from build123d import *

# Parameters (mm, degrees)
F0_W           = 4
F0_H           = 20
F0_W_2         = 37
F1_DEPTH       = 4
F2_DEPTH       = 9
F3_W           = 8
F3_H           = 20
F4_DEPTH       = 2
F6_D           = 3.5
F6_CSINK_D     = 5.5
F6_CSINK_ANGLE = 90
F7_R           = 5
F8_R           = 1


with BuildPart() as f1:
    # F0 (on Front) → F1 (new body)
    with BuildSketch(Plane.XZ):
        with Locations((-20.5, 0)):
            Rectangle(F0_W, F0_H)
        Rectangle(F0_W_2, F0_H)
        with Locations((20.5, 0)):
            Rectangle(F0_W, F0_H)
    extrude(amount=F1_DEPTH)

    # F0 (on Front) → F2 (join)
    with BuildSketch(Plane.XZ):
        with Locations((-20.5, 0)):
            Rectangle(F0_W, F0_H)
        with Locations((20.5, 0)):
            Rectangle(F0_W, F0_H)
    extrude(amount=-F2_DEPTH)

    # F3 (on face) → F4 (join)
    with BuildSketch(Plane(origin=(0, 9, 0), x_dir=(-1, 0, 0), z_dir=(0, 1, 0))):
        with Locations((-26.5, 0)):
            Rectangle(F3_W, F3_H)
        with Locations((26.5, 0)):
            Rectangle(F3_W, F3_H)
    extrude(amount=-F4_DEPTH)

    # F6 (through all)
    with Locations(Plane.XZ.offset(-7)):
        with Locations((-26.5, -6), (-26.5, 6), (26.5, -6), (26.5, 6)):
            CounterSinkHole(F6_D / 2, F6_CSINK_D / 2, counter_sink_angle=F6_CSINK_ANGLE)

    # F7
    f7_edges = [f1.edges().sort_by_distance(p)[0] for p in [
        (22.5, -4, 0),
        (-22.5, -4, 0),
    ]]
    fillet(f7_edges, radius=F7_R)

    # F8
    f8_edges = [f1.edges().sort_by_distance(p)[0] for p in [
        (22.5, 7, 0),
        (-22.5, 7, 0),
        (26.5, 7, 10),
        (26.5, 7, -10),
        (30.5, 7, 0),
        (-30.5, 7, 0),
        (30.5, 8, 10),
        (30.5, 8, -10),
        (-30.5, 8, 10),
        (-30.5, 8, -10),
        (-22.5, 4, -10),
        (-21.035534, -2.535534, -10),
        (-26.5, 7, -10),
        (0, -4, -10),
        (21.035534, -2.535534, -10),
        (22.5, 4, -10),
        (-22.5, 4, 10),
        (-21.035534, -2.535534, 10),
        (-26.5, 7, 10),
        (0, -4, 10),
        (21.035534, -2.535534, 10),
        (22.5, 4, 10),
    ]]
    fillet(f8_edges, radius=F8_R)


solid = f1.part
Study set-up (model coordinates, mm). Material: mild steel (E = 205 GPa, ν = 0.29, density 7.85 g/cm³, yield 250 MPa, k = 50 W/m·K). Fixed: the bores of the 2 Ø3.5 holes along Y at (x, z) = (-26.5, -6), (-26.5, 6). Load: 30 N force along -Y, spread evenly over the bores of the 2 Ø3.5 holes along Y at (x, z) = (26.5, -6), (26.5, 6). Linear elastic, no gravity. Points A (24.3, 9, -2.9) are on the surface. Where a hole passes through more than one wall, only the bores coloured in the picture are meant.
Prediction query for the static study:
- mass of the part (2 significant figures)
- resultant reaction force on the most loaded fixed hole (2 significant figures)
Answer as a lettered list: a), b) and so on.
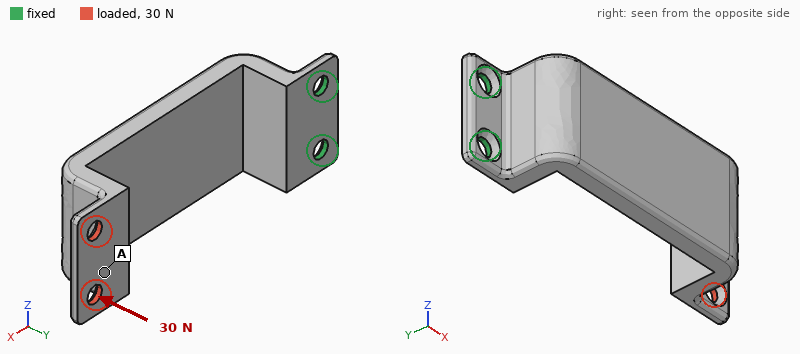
a) 42 g
b) 22 N
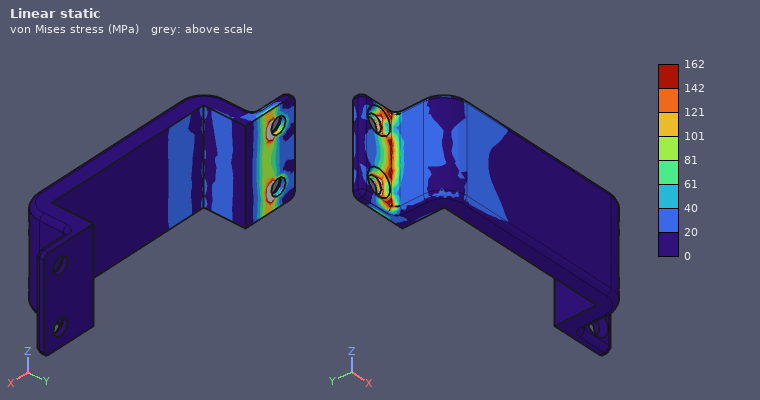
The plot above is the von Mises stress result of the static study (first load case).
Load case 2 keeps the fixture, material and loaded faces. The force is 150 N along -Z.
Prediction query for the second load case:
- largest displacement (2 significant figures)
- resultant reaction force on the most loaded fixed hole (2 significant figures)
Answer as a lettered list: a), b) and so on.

a) 0.16 mm
b) 560 N
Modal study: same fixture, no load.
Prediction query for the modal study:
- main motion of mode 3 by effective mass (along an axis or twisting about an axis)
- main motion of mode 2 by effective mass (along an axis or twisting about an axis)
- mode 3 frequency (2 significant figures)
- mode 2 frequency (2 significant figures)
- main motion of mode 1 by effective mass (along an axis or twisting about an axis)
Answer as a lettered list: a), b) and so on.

a) along X
b) along Z
c) 3100 Hz
d) 1600 Hz
e) along Y
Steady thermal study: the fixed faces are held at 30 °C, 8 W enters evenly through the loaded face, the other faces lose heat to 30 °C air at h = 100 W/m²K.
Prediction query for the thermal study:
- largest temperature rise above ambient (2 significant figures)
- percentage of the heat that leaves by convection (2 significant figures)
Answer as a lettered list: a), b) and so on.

a) 68 K
b) 86 %
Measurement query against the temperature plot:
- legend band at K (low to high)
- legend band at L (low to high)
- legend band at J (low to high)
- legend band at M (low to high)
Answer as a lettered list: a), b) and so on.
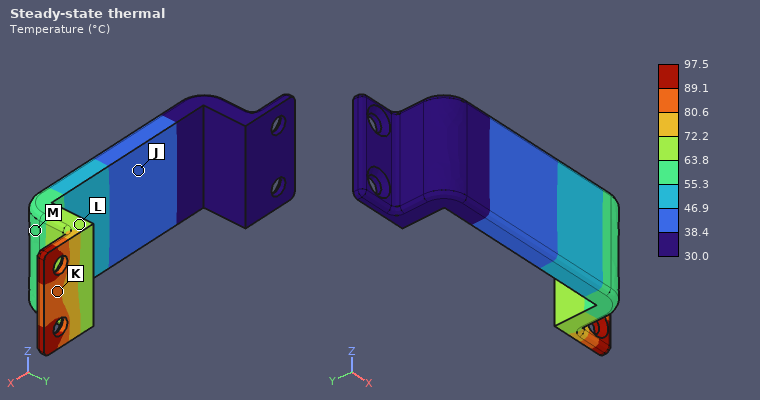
a) 80.6 to 89.1 °C
b) 63.8 to 72.2 °C
c) 38.4 to 46.9 °C
d) 55.3 to 63.8 °C
